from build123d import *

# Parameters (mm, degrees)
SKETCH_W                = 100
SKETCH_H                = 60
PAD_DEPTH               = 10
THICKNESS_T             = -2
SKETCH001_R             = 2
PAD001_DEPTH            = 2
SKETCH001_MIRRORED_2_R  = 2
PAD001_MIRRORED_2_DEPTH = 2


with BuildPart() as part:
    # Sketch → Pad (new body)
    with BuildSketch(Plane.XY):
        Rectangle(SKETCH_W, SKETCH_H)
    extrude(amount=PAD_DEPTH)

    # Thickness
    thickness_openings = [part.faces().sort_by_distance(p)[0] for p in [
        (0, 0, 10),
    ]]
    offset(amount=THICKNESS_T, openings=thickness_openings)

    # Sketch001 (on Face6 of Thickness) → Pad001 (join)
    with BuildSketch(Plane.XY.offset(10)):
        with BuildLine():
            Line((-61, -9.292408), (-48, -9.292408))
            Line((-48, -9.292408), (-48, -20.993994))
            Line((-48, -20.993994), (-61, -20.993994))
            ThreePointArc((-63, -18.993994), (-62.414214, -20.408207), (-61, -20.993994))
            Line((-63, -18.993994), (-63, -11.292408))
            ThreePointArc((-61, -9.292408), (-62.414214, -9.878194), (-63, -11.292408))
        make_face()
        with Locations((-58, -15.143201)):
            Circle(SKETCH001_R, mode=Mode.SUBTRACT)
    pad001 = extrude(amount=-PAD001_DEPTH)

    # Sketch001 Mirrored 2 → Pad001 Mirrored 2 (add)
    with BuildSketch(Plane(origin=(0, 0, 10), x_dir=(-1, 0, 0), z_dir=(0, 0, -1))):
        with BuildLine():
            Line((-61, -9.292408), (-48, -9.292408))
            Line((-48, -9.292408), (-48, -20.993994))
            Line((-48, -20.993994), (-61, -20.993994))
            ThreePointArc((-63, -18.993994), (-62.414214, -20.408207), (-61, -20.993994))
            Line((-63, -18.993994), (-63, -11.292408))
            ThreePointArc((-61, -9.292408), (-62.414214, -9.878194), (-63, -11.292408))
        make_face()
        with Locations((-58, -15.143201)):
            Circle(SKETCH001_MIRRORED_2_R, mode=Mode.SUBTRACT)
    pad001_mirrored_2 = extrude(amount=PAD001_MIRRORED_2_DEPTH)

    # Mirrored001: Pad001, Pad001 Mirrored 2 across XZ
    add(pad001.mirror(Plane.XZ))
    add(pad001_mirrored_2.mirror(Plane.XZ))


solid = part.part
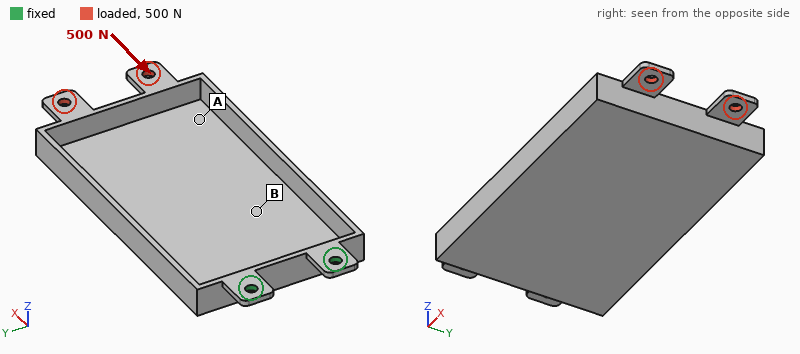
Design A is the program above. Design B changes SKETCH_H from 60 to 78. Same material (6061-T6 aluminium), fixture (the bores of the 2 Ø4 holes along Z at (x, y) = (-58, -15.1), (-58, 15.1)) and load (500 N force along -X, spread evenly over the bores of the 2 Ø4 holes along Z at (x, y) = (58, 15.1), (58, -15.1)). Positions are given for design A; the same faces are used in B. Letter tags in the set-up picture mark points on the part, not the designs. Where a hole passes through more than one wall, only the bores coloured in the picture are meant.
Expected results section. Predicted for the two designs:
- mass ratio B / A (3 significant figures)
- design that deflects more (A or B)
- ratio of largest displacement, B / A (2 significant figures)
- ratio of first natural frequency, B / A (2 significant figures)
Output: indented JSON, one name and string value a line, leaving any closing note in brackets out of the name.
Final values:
{
  "mass ratio B / A": "1.23",
  "design that deflects more": "B",
  "ratio of largest displacement, B / A": "1.5",
  "ratio of first natural frequency, B / A": "0.86"
}
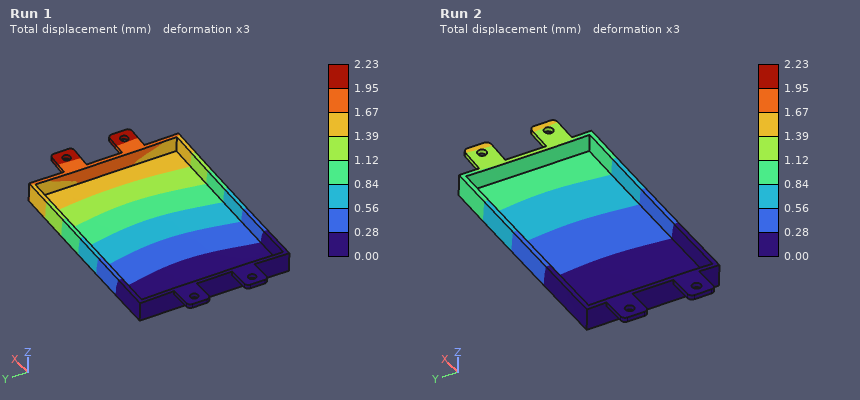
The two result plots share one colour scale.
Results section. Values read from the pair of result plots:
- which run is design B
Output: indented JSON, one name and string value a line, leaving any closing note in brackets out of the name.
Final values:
{
  "which run is design B": "Run 1"
}
